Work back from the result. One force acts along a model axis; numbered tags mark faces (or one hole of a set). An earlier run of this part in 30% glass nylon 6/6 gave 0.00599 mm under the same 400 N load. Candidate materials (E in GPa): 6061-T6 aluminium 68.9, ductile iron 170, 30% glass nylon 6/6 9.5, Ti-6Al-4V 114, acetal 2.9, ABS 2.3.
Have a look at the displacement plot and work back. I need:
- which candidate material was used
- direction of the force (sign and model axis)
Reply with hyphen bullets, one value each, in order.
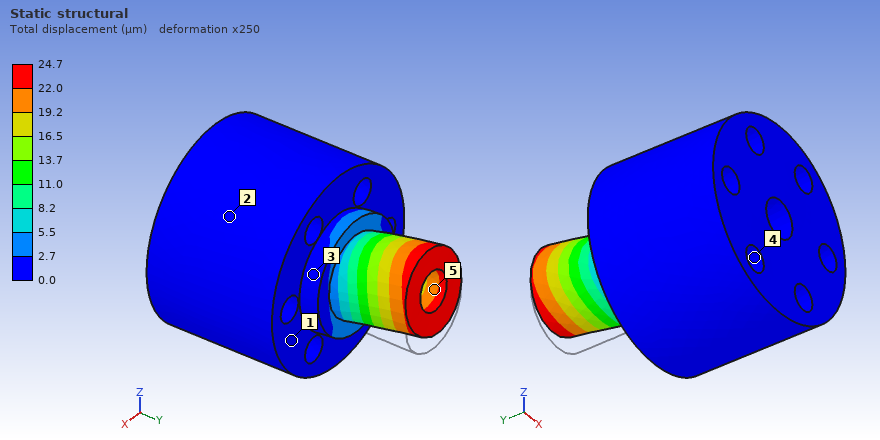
- ABS
- +Z
